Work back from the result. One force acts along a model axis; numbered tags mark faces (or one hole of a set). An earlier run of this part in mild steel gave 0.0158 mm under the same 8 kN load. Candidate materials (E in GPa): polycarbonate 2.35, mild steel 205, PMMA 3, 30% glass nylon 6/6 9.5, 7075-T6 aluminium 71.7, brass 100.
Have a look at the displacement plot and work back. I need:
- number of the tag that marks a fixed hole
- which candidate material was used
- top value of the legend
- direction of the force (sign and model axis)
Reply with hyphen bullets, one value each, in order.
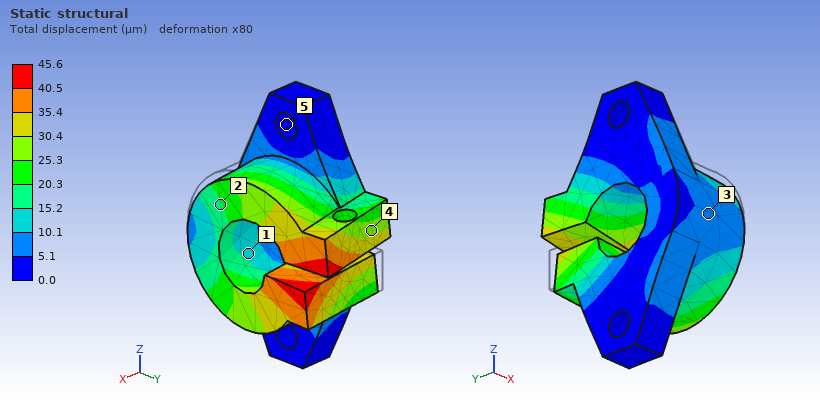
- 5
- 7075-T6 aluminium
- 45.6 µm
- -Z
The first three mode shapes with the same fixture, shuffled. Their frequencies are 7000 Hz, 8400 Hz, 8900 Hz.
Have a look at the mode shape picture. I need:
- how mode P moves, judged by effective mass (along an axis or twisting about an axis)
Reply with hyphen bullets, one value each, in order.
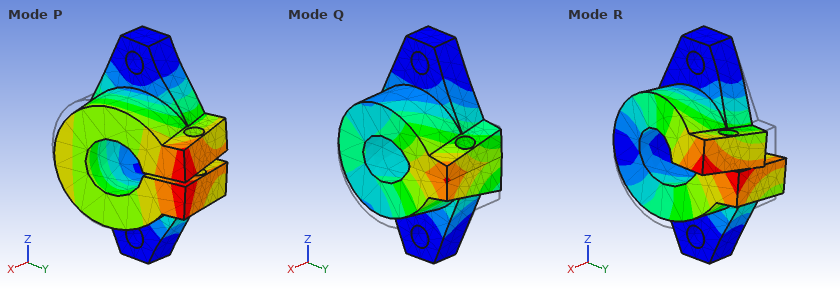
- along Y
